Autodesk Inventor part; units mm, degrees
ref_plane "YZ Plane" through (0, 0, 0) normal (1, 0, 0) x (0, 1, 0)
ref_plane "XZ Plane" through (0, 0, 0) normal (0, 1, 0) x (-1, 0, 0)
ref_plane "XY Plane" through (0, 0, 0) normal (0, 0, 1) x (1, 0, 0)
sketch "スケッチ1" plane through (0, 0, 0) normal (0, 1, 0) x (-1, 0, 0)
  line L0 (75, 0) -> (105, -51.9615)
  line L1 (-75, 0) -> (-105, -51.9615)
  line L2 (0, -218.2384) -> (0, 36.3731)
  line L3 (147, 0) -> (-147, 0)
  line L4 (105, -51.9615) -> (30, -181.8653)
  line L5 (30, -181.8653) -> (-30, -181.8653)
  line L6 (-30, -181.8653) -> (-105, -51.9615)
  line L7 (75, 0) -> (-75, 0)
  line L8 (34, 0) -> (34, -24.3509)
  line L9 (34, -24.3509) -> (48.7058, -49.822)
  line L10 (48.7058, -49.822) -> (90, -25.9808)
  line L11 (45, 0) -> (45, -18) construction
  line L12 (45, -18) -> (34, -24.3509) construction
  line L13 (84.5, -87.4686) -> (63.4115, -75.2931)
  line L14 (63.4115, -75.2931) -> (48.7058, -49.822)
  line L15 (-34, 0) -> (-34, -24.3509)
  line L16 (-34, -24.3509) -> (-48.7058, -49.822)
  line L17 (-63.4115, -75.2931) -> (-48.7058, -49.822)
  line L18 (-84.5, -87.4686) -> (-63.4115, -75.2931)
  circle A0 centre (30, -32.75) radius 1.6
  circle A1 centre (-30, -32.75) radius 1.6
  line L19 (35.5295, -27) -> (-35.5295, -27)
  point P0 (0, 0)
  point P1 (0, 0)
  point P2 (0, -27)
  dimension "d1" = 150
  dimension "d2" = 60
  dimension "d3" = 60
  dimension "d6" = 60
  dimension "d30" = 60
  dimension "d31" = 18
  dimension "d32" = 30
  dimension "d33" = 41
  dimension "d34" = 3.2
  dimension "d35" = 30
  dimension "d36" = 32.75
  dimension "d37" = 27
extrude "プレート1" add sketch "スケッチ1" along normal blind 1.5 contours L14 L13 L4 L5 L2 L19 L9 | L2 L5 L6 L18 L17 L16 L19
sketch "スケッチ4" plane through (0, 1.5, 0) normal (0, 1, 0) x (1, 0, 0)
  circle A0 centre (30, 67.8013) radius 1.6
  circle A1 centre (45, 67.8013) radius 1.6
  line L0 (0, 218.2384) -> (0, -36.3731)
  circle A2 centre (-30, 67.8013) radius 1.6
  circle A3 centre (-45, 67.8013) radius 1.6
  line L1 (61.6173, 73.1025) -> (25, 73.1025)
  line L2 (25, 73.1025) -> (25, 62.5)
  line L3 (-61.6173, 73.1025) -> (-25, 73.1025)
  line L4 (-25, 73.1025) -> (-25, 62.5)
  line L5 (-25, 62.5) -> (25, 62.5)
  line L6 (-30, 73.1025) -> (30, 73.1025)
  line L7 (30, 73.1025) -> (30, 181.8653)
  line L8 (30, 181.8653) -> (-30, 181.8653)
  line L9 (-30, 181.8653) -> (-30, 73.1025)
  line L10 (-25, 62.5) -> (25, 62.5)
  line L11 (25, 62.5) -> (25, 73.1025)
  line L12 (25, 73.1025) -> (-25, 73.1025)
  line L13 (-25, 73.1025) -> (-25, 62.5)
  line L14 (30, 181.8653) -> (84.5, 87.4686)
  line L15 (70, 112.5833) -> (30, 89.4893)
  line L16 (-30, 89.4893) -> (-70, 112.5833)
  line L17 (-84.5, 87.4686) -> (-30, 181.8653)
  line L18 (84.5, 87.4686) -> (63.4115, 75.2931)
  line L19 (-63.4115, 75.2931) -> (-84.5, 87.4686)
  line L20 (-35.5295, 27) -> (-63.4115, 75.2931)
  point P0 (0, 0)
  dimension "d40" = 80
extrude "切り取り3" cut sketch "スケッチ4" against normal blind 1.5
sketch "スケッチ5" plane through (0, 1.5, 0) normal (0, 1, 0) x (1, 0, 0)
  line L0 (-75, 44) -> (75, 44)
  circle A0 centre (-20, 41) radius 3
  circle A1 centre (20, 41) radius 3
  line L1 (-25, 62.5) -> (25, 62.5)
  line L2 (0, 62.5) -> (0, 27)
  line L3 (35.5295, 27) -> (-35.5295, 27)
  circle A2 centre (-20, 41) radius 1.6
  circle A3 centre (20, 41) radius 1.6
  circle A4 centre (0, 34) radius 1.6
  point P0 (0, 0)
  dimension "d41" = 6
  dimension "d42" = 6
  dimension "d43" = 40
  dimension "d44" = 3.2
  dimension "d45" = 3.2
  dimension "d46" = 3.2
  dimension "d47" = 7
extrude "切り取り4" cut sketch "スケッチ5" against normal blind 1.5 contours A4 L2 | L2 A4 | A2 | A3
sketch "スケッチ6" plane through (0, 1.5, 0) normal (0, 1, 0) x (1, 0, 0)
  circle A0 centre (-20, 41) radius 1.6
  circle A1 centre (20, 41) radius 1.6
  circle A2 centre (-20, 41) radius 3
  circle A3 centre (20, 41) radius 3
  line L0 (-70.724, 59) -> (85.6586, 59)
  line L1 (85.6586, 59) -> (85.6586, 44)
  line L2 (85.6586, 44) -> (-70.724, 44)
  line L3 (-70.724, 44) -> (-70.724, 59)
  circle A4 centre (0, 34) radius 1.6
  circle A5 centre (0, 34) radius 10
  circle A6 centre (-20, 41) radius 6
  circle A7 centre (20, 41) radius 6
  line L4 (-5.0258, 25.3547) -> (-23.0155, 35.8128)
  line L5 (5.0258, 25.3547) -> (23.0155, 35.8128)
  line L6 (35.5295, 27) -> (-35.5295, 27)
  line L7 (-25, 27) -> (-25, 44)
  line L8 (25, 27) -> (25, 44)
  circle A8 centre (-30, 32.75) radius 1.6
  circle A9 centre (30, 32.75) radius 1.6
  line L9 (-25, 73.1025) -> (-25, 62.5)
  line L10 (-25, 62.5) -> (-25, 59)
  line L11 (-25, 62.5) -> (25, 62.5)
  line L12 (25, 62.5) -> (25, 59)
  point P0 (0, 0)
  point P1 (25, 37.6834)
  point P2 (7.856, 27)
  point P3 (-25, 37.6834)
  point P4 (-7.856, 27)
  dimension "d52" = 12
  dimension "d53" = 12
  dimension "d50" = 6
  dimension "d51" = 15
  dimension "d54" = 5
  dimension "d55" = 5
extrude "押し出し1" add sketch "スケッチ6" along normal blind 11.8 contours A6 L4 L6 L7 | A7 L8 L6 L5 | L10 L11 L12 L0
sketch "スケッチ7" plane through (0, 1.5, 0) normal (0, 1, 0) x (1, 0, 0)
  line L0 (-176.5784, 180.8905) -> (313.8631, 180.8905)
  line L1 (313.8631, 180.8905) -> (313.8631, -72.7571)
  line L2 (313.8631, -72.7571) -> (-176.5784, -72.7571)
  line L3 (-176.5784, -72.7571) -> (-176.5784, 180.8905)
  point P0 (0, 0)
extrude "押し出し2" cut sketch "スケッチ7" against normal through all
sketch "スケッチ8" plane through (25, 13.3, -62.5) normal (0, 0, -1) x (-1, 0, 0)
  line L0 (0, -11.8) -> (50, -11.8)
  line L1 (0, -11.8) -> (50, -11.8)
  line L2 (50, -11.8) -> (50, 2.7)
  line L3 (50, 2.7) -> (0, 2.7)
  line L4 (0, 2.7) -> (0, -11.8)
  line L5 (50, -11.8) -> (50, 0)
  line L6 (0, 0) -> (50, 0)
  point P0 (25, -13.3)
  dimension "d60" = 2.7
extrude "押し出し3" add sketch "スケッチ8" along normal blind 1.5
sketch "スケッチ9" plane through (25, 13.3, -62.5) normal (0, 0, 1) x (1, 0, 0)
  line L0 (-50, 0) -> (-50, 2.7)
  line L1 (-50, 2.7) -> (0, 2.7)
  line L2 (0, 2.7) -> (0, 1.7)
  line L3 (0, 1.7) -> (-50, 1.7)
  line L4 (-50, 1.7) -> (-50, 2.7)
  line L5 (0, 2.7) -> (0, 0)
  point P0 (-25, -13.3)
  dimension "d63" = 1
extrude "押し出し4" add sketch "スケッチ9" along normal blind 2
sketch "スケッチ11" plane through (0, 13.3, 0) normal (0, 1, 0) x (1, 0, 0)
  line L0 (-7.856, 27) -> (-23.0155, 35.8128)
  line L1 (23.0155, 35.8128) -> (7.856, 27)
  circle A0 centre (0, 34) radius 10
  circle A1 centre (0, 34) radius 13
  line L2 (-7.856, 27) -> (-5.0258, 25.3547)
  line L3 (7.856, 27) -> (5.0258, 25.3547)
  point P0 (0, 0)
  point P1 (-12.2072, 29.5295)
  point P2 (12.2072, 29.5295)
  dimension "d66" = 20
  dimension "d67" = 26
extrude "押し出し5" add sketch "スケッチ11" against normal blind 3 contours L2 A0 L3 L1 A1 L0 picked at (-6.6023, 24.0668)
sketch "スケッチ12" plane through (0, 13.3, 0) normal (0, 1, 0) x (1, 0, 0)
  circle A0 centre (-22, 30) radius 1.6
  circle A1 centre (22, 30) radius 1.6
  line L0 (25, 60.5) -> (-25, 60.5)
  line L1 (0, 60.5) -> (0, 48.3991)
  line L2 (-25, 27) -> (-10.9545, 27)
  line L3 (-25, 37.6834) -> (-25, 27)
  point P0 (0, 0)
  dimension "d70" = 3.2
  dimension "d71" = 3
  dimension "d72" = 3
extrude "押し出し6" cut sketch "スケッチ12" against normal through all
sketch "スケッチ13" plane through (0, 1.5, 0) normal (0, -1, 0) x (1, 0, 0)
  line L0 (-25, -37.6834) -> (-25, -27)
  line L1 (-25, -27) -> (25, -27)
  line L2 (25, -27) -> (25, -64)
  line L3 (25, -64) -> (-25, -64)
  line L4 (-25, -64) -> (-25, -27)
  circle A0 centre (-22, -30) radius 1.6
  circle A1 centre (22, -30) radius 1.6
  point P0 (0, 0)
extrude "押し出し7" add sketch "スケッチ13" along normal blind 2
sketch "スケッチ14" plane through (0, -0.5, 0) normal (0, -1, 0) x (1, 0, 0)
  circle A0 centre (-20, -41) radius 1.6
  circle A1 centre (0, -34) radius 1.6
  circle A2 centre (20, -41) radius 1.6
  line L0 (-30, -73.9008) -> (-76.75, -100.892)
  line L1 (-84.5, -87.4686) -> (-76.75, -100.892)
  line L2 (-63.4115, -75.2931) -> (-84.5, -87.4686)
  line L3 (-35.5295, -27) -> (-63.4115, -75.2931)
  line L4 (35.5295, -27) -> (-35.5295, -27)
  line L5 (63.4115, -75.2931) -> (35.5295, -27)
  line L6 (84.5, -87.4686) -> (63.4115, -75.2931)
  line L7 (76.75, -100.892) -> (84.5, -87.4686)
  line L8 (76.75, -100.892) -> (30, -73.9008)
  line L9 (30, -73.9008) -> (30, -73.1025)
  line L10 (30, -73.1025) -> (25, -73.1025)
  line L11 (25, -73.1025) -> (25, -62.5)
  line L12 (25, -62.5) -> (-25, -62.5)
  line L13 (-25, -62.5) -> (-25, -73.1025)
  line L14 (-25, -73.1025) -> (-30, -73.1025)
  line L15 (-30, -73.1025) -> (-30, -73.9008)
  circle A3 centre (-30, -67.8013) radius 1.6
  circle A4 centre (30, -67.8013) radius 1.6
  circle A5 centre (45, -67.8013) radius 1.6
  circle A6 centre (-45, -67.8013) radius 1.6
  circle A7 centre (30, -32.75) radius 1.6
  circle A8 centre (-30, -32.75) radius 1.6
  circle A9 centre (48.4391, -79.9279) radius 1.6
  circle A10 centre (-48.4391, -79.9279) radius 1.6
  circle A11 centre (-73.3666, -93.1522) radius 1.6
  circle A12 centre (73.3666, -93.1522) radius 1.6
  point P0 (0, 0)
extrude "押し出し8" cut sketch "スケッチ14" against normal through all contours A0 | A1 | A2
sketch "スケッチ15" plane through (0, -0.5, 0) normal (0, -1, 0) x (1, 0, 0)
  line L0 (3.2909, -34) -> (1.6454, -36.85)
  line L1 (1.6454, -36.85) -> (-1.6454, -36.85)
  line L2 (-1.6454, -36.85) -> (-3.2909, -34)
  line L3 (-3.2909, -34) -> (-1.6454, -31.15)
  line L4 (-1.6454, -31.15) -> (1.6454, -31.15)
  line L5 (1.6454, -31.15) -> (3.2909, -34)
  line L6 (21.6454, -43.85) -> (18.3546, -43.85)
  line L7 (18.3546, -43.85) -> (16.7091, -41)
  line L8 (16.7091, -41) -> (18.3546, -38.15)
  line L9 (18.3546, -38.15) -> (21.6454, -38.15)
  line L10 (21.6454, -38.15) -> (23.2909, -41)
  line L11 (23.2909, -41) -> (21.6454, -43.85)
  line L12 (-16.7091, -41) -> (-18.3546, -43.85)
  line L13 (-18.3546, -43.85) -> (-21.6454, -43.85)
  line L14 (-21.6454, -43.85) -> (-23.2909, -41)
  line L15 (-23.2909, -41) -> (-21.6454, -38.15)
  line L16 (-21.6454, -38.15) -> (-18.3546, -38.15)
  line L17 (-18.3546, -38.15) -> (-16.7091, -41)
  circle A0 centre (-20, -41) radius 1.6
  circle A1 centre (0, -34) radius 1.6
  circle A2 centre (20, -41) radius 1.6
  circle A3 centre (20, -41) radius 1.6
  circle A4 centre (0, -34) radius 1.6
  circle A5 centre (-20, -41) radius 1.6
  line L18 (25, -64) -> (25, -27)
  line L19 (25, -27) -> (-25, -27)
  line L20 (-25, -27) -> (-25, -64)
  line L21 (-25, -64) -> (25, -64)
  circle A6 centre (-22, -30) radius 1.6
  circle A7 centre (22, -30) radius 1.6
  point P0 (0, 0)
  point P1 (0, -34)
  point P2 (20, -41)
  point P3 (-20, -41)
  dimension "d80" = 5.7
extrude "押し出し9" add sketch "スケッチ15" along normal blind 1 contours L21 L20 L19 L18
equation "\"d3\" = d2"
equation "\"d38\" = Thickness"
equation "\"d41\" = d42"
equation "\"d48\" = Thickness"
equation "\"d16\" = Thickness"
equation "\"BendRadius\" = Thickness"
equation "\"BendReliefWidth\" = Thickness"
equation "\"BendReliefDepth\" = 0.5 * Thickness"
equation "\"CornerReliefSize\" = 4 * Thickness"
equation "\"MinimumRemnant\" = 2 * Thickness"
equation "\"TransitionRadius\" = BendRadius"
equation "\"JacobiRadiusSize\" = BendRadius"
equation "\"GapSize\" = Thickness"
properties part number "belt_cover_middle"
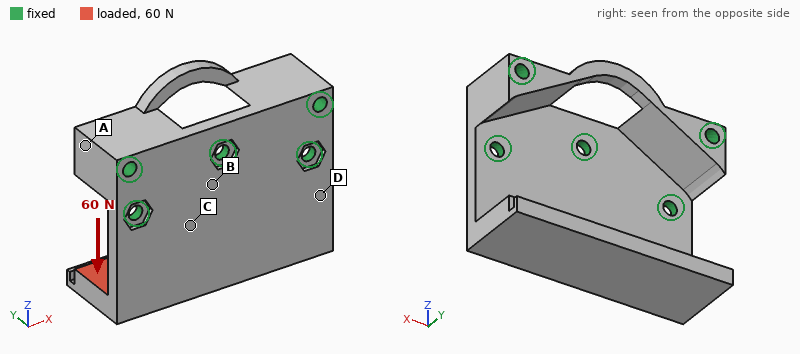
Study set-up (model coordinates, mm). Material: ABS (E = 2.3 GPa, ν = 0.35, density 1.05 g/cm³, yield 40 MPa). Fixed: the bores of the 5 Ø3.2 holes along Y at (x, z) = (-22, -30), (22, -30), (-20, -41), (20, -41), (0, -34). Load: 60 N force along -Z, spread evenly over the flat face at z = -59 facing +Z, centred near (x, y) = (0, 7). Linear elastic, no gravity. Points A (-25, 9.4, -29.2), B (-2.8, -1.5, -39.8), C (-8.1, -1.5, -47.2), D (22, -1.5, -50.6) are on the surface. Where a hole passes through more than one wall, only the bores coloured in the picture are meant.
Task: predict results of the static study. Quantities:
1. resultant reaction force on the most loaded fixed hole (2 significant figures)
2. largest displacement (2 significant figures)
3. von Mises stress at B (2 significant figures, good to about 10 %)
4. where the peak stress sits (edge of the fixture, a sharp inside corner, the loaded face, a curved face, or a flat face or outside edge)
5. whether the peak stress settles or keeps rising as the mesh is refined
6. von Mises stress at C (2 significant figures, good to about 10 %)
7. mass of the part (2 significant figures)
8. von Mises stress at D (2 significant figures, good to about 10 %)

31 N
0.78 mm
2.9 MPa
edge of the fixture
keeps rising
4.7 MPa
11 g
5.5 MPa
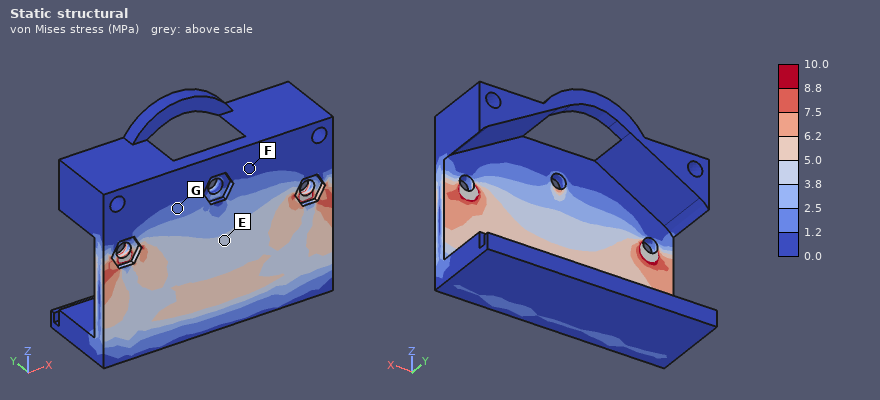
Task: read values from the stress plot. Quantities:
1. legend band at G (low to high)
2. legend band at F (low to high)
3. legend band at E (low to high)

1.2 to 2.5 MPa
0.0 to 1.2 MPa
3.8 to 5.0 MPa
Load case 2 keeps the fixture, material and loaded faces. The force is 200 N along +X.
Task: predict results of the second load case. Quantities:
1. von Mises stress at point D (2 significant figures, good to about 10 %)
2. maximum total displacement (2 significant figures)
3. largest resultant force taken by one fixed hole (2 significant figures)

5.6 MPa
0.78 mm
100 N
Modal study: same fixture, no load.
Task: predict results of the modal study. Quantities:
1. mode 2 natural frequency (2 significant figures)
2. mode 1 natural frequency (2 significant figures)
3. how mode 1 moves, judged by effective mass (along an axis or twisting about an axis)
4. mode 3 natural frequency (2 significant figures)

1100 Hz
510 Hz
along Y
2100 Hz
